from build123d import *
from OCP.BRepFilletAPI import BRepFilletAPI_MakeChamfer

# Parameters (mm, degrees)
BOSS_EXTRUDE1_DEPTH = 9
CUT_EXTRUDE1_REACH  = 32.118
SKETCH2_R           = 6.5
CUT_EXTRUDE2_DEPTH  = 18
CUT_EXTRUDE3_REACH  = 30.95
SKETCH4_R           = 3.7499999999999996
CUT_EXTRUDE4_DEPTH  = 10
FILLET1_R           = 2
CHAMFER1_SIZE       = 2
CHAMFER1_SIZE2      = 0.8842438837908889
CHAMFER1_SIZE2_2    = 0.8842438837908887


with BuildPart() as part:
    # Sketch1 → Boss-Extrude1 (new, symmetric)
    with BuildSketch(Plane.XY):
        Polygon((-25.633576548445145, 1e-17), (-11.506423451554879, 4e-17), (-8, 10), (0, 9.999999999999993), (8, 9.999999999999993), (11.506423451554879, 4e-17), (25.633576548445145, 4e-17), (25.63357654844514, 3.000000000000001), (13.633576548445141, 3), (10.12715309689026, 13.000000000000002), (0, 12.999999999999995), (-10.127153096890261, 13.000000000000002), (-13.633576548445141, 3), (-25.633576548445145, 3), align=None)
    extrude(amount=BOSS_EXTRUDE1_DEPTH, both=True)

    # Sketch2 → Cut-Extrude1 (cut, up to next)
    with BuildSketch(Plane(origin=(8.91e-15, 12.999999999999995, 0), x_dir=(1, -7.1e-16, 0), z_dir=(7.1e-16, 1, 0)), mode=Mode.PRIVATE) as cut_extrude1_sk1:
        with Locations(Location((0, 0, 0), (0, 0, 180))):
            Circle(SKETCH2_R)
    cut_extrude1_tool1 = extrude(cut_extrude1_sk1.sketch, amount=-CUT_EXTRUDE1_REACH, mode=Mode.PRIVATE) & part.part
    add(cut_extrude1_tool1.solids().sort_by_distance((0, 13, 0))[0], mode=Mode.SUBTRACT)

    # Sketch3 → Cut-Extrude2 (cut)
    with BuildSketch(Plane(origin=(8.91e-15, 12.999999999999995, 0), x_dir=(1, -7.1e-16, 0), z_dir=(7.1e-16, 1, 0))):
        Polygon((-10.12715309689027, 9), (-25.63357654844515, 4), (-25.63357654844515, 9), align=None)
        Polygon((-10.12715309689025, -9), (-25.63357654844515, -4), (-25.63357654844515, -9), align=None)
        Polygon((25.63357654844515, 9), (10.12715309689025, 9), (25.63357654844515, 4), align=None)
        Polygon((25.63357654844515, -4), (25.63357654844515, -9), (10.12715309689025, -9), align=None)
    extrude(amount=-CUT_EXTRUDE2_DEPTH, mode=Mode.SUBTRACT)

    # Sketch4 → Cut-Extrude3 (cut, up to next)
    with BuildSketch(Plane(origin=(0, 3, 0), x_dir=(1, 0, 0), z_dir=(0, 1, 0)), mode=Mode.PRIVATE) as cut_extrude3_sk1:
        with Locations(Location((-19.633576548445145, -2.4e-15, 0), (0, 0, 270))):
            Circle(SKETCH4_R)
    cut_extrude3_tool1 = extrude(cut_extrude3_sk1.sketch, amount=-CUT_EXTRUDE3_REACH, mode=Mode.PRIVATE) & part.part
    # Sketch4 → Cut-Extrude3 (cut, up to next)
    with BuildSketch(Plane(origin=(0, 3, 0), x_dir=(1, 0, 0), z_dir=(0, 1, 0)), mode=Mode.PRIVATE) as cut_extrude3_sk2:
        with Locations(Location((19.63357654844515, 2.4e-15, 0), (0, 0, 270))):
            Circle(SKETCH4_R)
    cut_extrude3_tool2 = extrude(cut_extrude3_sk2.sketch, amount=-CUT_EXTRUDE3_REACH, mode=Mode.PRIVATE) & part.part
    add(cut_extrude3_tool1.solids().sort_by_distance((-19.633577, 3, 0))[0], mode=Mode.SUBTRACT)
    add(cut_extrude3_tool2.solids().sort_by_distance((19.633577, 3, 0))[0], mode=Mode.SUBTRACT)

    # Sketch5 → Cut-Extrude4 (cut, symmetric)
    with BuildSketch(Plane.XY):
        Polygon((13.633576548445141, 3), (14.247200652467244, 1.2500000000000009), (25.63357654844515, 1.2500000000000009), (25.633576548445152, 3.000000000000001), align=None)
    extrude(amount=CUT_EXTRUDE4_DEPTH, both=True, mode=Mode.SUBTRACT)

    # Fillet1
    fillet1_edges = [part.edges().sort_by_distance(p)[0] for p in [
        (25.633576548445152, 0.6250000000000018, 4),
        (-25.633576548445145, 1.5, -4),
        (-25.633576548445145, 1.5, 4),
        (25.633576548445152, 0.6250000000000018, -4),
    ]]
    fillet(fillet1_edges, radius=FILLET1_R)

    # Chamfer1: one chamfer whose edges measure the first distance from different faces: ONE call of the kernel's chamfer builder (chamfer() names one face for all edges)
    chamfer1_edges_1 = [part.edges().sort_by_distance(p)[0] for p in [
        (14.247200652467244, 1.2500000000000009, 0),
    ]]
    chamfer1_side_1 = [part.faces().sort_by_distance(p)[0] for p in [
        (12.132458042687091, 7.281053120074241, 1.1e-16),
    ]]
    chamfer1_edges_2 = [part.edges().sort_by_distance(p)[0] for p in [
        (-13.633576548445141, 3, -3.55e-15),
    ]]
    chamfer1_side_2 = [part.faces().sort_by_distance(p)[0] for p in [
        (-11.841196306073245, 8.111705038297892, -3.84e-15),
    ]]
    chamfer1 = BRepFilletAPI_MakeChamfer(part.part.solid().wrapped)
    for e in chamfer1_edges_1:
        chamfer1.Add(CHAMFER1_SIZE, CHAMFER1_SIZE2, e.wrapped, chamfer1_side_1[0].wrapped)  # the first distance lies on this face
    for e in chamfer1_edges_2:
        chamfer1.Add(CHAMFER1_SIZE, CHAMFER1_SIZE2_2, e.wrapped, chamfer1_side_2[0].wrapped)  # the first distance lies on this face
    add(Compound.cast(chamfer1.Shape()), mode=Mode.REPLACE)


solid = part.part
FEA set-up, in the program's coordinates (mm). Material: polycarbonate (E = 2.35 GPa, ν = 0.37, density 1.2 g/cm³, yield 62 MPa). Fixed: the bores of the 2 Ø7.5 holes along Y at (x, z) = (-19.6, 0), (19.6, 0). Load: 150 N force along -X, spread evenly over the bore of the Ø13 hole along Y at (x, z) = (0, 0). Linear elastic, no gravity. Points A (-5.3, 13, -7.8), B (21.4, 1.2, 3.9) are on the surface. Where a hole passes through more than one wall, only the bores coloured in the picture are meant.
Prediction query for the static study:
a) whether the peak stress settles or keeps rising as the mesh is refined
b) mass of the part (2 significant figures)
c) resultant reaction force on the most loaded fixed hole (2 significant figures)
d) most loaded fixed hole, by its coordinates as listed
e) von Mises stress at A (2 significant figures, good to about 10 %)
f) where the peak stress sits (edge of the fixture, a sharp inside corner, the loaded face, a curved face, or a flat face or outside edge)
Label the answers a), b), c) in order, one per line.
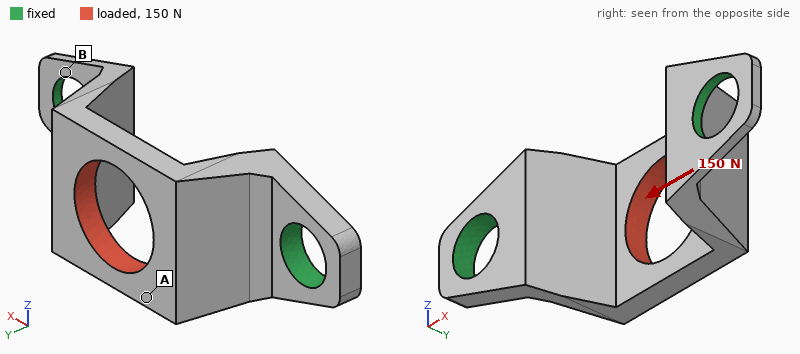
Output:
a) keeps rising
b) 2.7 g
c) 99 N
d) (-19.6, 0)
e) 14 MPa
f) a sharp inside corner
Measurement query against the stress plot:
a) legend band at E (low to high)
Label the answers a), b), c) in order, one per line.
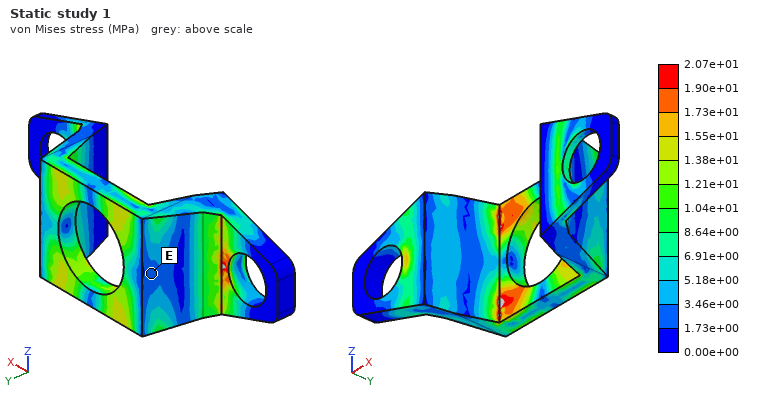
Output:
a) 1.73e+00 to 3.46e+00 MPa
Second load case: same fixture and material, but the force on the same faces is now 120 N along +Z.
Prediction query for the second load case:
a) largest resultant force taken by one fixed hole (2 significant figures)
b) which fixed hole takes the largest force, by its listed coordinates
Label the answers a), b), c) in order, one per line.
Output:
a) 77 N
b) (-19.6, 0)
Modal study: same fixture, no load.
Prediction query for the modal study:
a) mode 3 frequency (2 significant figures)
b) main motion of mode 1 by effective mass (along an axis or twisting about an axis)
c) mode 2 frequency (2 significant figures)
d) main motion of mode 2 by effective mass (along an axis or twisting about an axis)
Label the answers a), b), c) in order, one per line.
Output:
a) 4100 Hz
b) along Z
c) 3300 Hz
d) along X
